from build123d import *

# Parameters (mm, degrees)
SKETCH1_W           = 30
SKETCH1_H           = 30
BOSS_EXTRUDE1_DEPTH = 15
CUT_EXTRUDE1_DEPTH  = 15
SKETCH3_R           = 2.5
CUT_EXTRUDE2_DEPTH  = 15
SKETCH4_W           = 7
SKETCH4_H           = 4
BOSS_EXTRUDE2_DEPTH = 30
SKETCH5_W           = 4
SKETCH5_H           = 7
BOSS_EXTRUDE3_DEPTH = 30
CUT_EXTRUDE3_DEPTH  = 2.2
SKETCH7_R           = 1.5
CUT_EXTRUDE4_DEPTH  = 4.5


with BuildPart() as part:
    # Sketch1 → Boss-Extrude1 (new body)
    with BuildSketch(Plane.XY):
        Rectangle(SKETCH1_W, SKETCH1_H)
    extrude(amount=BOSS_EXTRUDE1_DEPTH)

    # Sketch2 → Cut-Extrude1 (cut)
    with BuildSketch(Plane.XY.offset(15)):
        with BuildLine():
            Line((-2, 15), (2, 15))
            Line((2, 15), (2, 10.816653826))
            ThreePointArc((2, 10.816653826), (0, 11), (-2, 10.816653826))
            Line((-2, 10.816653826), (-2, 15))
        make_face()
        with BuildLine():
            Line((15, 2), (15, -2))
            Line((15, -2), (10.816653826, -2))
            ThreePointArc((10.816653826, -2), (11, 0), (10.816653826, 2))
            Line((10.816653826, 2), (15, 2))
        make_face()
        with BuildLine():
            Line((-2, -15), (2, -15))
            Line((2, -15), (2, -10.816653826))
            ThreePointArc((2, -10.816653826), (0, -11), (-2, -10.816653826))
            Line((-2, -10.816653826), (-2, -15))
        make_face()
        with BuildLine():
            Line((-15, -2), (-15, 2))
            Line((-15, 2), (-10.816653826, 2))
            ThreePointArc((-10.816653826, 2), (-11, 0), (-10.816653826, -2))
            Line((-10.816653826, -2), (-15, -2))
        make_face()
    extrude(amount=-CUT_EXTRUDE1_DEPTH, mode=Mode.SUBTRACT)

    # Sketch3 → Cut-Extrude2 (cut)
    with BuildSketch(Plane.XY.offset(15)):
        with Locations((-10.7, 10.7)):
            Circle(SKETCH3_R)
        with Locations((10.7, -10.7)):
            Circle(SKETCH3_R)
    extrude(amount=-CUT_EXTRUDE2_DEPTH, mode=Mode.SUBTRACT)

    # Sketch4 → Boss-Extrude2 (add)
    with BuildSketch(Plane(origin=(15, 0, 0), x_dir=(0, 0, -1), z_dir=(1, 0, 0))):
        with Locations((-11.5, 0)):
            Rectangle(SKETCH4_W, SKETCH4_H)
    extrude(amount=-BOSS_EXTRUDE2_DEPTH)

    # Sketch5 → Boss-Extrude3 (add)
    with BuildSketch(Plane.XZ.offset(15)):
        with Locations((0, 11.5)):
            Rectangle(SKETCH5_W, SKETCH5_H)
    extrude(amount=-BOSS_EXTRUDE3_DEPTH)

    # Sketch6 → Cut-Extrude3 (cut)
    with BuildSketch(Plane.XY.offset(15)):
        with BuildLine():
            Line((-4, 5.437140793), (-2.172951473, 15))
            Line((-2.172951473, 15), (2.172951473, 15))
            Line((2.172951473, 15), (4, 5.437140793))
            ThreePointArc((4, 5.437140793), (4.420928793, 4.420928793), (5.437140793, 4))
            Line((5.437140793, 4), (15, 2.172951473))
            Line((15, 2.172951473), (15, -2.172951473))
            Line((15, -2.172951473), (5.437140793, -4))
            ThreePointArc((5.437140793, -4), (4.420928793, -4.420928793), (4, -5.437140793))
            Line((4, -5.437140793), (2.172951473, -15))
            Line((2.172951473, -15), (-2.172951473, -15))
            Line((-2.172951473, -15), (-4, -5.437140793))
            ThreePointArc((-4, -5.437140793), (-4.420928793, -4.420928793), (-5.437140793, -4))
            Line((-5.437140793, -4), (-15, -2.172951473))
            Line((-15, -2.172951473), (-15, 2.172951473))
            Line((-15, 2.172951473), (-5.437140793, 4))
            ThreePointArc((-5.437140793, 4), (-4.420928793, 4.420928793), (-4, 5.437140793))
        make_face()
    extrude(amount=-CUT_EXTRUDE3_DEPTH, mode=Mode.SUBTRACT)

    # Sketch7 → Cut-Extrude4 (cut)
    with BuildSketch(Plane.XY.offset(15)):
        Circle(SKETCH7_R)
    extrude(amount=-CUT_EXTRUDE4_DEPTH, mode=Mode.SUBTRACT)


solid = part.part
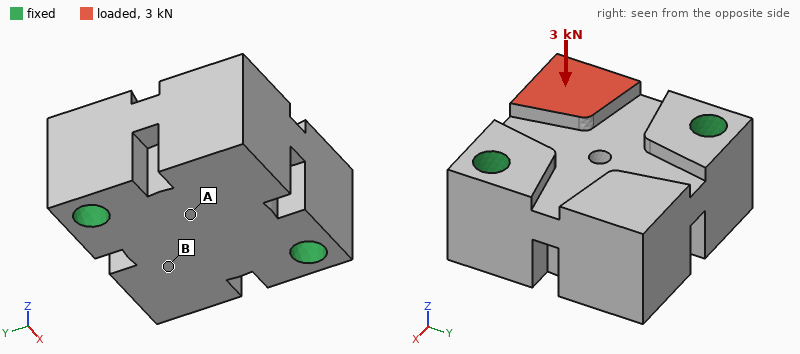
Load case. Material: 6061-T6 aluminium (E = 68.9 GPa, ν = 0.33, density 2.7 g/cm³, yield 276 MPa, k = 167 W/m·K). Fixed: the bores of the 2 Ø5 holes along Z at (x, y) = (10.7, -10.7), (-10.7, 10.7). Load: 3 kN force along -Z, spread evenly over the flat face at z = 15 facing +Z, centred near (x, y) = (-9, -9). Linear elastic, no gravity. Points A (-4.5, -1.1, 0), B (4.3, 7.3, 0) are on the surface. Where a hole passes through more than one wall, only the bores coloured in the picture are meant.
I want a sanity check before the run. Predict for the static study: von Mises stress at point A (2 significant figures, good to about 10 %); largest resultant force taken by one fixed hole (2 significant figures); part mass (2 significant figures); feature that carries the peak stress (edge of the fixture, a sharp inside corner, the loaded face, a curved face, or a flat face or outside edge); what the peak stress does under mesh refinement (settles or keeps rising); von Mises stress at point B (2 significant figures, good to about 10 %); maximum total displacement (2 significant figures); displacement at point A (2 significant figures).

36 MPa
1.5 kN
31 g
edge of the fixture
keeps rising
10 MPa
44 µm
12 µm
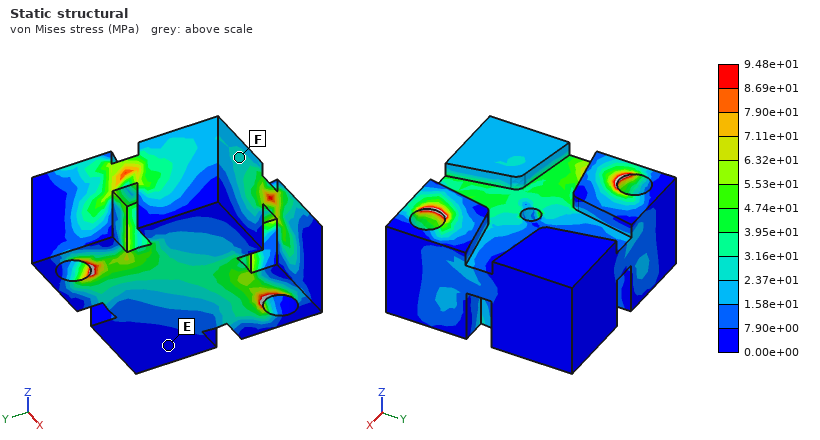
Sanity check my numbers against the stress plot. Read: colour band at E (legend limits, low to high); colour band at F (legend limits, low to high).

0.00e+00 to 7.90e+00 MPa
2.37e+01 to 3.16e+01 MPa
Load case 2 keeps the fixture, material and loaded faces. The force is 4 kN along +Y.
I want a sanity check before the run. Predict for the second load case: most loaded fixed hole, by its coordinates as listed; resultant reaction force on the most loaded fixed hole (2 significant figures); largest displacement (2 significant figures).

(-10.7, 10.7)
3.3 kN
41 µm
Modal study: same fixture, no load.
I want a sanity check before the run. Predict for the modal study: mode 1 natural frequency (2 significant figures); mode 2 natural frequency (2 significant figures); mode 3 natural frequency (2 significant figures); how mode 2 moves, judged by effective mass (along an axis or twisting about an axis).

18 kHz
24 kHz
34 kHz
along Z
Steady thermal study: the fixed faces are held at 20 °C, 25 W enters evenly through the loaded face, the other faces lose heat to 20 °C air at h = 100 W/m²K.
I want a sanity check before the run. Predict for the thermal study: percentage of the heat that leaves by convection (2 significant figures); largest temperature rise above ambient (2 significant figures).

4.2 %
15 K
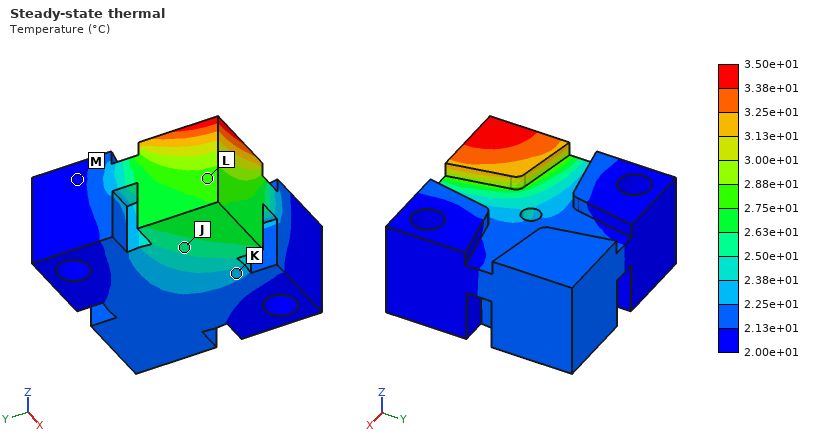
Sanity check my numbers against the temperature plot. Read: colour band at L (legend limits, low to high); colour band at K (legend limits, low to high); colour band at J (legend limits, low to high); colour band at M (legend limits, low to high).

2.75e+01 to 2.88e+01 °C
2.25e+01 to 2.38e+01 °C
2.50e+01 to 2.63e+01 °C
2.00e+01 to 2.13e+01 °C
